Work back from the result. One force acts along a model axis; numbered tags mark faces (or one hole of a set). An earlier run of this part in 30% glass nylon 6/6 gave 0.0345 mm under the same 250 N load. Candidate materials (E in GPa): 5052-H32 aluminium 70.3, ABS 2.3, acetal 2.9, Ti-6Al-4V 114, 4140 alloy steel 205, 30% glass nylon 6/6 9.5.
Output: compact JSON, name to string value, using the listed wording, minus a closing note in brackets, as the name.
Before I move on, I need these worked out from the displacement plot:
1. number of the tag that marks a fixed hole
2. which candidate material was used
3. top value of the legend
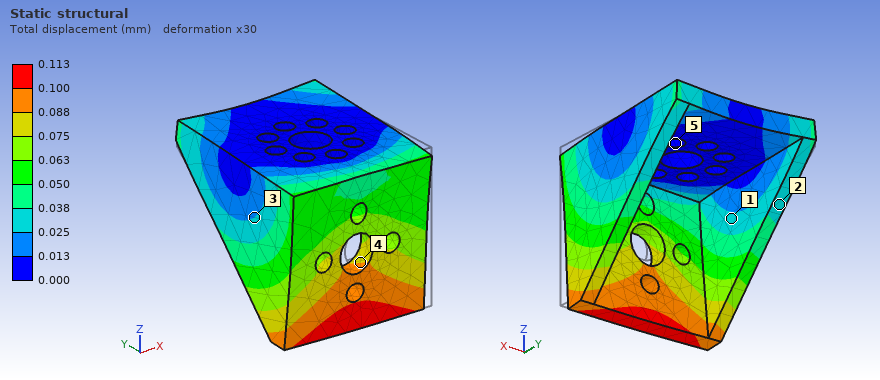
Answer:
{"number of the tag that marks a fixed hole": "5", "which candidate material was used": "acetal", "top value of the legend": "0.113 mm"}
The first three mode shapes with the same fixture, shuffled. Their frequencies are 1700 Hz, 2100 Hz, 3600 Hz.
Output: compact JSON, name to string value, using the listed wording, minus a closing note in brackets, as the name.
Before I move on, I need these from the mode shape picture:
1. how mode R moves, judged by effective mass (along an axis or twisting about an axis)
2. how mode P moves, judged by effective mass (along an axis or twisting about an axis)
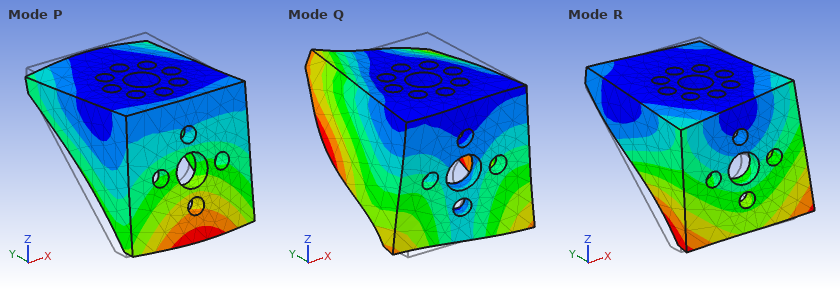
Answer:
{"how mode R moves, judged by effective mass": "along X", "how mode P moves, judged by effective mass": "along Y"}
